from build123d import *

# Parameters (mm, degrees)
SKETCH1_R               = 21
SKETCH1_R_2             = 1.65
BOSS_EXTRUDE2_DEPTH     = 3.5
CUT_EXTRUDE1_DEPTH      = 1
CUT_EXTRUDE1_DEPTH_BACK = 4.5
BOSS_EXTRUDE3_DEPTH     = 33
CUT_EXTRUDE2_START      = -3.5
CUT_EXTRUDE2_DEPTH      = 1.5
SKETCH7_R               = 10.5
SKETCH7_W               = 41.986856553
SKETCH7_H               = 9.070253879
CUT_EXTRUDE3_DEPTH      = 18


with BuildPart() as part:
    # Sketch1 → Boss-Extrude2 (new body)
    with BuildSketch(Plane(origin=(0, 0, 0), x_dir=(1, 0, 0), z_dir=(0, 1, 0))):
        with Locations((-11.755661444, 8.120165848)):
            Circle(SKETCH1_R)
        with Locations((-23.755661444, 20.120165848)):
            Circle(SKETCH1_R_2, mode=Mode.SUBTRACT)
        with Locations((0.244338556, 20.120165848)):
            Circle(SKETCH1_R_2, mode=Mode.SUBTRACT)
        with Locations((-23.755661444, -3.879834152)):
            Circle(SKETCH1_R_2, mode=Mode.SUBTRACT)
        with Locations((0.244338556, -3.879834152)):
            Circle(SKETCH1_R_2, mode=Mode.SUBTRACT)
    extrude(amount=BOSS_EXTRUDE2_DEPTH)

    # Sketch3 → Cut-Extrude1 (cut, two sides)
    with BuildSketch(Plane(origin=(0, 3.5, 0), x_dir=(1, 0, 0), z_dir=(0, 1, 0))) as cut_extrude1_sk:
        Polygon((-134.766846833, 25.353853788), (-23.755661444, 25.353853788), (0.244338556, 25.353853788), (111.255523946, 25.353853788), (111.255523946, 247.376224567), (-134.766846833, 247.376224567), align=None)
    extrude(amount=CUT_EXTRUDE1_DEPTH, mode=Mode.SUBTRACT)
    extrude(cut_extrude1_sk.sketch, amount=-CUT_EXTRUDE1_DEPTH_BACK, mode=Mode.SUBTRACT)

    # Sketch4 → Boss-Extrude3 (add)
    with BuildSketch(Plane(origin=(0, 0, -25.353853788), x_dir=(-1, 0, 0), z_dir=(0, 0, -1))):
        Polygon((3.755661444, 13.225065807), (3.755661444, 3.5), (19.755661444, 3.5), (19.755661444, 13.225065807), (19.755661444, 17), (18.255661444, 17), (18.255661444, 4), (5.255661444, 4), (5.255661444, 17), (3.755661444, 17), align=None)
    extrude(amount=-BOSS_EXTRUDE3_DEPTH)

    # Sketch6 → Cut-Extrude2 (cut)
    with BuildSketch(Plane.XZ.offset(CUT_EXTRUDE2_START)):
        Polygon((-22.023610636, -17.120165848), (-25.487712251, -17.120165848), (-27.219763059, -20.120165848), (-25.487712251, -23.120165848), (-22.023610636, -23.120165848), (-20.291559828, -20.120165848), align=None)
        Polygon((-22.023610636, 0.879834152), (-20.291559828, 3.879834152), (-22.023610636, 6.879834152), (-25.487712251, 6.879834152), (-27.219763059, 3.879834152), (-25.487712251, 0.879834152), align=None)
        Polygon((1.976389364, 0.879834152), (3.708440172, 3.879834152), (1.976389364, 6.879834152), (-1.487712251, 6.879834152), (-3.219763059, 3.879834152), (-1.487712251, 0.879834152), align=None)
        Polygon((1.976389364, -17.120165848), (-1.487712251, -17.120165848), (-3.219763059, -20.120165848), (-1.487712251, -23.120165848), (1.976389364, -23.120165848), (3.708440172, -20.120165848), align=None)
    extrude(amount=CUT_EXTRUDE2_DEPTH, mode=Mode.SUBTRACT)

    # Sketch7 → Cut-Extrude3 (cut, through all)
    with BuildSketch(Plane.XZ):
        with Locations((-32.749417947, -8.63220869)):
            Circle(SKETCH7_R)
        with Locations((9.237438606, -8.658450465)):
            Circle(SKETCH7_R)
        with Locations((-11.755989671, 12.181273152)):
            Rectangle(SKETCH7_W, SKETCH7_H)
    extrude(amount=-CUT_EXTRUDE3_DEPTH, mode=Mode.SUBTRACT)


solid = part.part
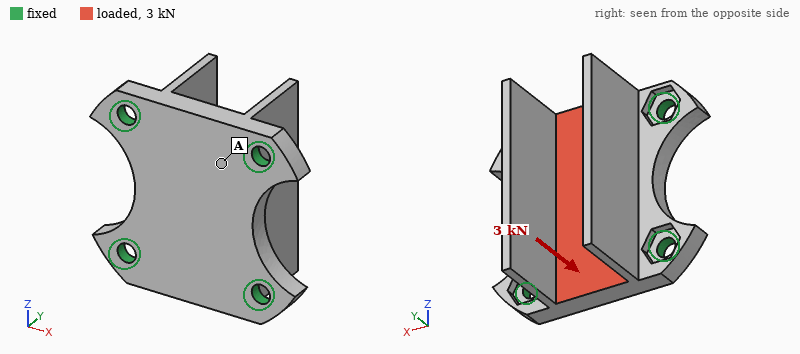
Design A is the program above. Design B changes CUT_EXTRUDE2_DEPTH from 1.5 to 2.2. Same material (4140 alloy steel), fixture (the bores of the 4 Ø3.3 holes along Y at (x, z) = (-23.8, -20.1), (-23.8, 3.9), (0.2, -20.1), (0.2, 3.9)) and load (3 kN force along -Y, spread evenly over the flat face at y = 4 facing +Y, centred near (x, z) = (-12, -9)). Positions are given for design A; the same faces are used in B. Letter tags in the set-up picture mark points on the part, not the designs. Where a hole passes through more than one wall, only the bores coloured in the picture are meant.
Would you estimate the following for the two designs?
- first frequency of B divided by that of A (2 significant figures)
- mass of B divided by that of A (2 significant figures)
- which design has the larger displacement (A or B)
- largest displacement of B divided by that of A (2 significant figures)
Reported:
1.00
0.99
B
1.1
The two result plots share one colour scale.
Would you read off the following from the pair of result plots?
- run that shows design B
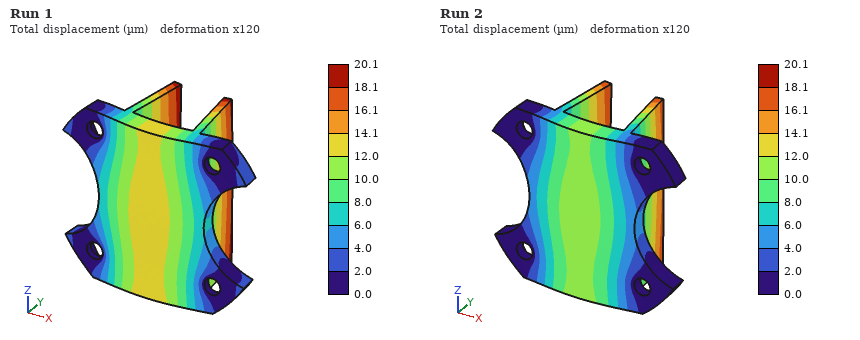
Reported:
Run 1
